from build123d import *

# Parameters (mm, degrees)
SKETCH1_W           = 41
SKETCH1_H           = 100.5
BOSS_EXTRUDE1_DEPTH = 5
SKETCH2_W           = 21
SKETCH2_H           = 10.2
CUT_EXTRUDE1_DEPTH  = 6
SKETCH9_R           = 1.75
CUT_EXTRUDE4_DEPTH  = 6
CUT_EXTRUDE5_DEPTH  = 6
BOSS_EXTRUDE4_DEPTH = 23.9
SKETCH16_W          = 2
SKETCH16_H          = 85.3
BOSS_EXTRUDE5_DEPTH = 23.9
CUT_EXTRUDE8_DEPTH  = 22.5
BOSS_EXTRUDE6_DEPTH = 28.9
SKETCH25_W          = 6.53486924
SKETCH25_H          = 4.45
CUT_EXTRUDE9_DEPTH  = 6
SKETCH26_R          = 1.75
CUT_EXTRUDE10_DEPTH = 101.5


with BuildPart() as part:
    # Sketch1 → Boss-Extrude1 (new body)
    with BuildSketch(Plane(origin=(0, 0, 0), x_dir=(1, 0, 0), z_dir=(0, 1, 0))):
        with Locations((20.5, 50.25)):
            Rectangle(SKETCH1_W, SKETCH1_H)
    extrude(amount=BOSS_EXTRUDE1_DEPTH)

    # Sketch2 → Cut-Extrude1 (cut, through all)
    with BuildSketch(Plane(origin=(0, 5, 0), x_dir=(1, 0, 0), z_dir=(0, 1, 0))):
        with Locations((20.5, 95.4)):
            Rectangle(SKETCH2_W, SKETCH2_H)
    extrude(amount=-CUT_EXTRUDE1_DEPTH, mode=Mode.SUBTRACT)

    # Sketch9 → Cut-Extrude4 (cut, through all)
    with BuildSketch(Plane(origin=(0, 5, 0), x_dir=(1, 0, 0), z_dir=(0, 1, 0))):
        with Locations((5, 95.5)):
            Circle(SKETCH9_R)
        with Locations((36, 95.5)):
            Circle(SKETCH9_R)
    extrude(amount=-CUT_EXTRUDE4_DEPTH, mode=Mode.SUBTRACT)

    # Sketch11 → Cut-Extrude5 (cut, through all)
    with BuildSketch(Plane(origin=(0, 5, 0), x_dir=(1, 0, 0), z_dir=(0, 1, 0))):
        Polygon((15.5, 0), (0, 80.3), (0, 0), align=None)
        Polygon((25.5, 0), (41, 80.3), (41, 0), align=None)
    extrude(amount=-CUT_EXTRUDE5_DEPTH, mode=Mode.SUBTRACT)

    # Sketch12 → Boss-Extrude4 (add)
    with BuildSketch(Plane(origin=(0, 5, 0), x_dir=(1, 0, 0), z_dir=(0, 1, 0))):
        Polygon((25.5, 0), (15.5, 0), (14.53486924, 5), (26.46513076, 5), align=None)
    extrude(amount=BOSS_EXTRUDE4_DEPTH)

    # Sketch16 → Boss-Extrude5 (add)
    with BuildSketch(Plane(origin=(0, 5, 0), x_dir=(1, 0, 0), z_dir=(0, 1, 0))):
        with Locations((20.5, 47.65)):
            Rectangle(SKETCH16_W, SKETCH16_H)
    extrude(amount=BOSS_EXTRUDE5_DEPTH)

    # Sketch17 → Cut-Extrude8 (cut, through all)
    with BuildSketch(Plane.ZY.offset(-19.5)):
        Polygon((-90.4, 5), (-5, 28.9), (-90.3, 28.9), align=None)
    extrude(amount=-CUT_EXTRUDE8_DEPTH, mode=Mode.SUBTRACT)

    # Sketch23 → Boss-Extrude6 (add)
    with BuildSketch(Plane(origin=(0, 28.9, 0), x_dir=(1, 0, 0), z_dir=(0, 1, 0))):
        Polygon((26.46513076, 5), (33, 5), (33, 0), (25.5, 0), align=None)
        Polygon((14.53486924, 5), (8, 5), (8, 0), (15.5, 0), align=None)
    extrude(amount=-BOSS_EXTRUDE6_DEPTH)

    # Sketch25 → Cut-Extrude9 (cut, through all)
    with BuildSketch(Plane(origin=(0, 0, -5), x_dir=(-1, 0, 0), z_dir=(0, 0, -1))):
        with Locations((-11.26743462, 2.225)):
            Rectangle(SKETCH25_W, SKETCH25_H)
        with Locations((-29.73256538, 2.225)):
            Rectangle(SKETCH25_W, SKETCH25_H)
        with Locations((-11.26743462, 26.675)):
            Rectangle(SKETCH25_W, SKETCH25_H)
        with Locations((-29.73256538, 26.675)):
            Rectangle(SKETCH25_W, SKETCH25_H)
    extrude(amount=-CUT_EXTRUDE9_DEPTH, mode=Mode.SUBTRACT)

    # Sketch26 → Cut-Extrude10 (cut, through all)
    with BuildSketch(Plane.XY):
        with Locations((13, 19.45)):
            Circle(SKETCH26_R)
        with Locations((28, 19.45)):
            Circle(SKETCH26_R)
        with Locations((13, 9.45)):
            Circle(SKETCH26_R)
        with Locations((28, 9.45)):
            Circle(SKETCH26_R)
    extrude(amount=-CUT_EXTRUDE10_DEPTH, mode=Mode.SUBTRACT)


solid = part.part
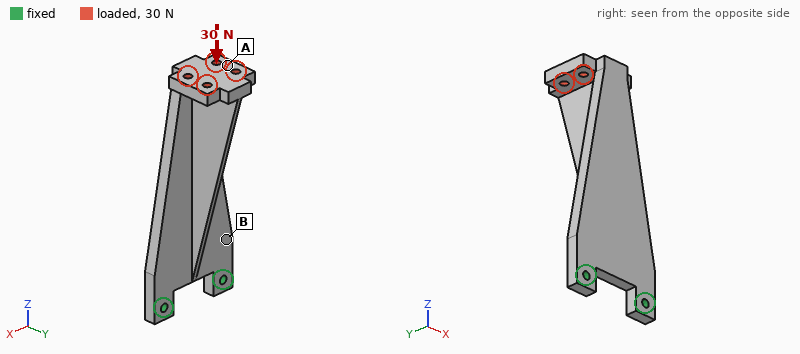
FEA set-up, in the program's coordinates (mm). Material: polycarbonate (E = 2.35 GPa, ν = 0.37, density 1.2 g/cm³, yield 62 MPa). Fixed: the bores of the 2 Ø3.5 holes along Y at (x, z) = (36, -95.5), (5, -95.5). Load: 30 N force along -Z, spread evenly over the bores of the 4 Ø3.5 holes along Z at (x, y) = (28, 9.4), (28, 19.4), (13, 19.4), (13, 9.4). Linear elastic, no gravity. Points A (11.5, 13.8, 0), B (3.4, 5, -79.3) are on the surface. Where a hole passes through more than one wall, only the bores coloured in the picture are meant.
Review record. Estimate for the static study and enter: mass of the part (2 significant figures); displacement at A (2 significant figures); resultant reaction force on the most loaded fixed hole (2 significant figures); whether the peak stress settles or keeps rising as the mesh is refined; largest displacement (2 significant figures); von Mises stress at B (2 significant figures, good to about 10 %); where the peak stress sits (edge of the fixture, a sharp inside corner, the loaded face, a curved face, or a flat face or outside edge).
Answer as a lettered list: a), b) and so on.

a) 21 g
b) 1.3 mm
c) 16 N
d) keeps rising
e) 1.3 mm
f) 2.2 MPa
g) edge of the fixture
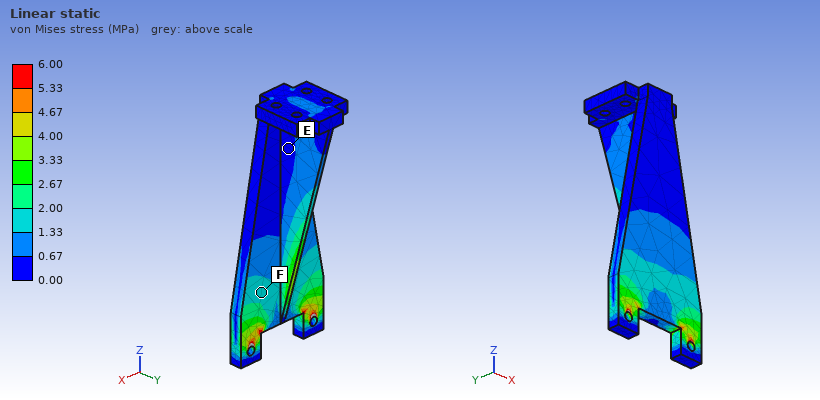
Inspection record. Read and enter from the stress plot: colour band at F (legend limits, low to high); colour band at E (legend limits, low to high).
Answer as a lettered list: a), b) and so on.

a) 1.33 to 2.00 MPa
b) 0.00 to 0.67 MPa
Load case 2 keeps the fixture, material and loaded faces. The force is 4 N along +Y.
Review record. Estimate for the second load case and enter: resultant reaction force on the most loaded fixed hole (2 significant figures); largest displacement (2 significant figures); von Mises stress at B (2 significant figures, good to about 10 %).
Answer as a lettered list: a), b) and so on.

a) 2.2 N
b) 1.2 mm
c) 1.8 MPa
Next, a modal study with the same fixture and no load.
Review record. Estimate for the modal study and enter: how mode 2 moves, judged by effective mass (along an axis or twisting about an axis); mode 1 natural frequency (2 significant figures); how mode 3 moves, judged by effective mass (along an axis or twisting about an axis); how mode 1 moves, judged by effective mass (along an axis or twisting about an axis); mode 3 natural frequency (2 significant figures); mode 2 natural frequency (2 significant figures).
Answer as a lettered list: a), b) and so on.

a) along X
b) 110 Hz
c) along X
d) along Y
e) 1000 Hz
f) 430 Hz
